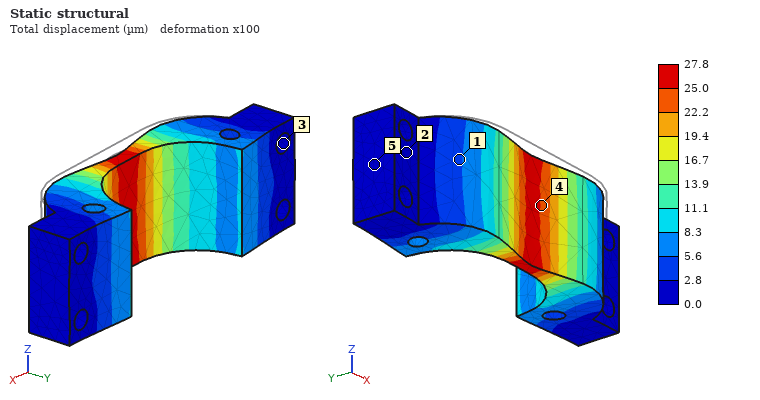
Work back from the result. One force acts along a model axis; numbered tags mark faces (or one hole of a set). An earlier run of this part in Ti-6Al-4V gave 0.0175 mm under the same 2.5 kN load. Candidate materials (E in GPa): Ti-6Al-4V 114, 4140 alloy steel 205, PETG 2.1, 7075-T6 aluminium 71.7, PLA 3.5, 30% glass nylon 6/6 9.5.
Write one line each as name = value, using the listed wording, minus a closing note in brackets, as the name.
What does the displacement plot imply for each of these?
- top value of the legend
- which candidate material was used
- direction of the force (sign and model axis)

top value of the legend = 27.8 µm
which candidate material was used = 7075-T6 aluminium
direction of the force = +Y
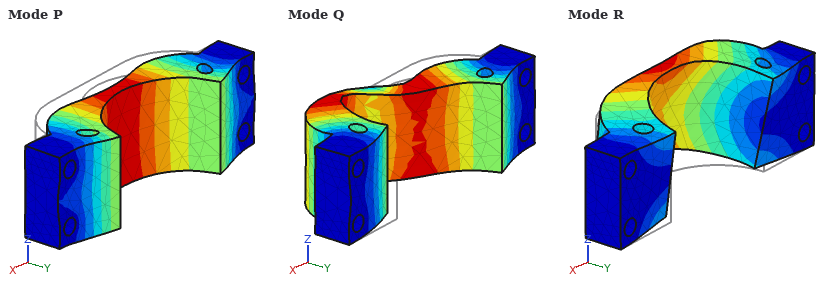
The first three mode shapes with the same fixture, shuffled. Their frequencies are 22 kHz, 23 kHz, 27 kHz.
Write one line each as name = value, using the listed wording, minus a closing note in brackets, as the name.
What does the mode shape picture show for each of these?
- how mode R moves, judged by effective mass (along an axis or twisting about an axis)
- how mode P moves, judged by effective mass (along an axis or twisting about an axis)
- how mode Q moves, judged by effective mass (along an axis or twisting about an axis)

how mode R moves, judged by effective mass = along Z
how mode P moves, judged by effective mass = along Y
how mode Q moves, judged by effective mass = along X
